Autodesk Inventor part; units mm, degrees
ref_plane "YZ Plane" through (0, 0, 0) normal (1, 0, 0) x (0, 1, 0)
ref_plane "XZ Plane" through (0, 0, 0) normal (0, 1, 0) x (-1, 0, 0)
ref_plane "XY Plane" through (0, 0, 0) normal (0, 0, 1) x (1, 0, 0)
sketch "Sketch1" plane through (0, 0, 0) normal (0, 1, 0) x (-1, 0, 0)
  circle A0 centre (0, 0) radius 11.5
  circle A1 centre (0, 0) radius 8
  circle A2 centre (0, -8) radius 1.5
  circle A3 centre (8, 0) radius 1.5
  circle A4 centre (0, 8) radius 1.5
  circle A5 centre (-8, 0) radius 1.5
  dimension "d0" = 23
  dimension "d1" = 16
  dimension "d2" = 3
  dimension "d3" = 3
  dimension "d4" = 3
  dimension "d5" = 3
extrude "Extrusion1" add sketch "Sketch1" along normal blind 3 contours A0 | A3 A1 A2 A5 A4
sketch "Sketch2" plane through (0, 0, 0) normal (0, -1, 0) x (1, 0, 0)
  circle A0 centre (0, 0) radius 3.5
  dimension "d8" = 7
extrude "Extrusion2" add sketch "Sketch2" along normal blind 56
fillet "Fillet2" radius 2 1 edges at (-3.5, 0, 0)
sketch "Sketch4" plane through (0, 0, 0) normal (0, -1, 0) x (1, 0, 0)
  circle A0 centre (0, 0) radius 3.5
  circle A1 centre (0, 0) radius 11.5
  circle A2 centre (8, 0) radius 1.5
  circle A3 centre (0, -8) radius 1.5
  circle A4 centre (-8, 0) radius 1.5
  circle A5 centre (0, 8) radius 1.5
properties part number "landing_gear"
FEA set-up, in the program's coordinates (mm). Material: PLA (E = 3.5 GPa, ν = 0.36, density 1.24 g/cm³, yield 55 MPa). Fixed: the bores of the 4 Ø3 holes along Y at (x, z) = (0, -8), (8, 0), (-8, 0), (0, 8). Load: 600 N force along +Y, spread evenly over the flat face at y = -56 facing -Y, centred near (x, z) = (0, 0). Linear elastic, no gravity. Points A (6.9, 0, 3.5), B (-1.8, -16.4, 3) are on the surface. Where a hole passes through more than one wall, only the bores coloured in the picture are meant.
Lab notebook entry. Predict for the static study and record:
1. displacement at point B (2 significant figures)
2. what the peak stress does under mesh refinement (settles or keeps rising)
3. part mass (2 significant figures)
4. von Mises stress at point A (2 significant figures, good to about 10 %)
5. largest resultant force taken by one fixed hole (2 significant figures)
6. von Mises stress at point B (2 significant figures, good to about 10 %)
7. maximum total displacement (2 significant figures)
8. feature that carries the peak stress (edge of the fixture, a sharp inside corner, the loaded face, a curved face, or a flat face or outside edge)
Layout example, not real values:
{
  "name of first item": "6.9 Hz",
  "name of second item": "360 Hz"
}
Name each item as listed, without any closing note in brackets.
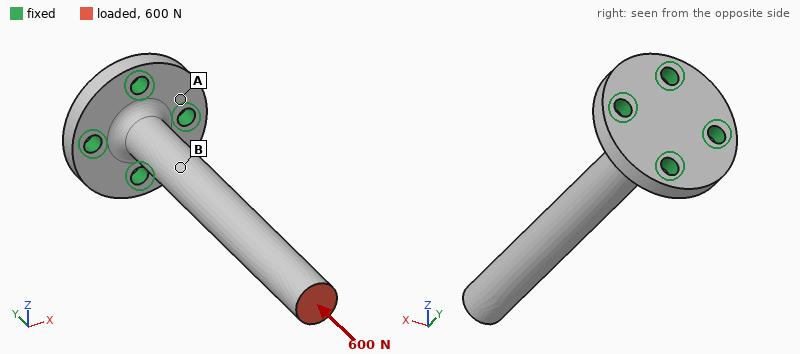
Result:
{
  "displacement at point B": "0.11 mm",
  "what the peak stress does under mesh refinement": "keeps rising",
  "part mass": "4.1 g",
  "von Mises stress at point A": "4.2 MPa",
  "largest resultant force taken by one fixed hole": "160 N",
  "von Mises stress at point B": "16 MPa",
  "maximum total displacement": "0.29 mm",
  "feature that carries the peak stress": "edge of the fixture"
}
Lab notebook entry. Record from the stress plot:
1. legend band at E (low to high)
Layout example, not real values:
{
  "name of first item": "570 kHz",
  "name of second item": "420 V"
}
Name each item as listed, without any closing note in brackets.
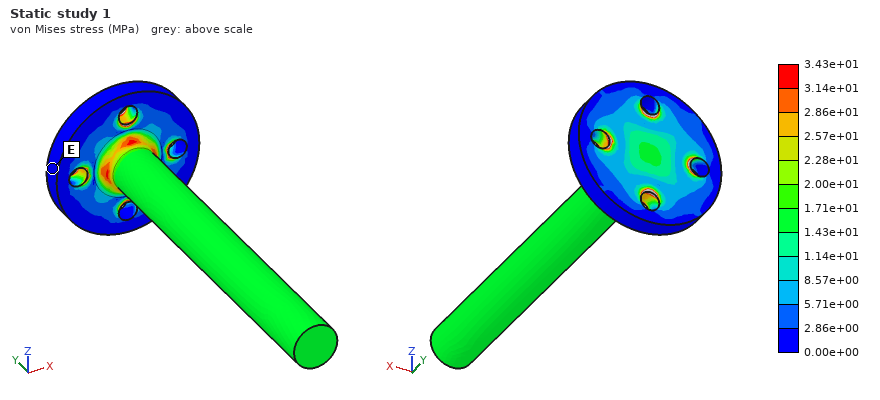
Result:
{
  "legend band at E": "0.00e+00 to 2.86e+00 MPa"
}
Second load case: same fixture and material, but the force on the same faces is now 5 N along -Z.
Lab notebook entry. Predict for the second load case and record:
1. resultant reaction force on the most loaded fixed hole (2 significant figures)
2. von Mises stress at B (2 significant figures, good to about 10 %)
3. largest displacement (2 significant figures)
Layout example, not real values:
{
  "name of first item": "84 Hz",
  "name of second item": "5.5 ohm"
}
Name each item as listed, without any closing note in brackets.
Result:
{
  "resultant reaction force on the most loaded fixed hole": "21 N",
  "von Mises stress at B": "5.0 MPa",
  "largest displacement": "0.76 mm"
}
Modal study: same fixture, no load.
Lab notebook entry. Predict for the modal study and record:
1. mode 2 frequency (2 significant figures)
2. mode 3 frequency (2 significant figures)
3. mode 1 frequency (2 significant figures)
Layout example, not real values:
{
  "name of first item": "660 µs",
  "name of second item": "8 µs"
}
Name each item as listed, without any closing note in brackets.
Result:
{
  "mode 2 frequency": "500 Hz",
  "mode 3 frequency": "3000 Hz",
  "mode 1 frequency": "500 Hz"
}
